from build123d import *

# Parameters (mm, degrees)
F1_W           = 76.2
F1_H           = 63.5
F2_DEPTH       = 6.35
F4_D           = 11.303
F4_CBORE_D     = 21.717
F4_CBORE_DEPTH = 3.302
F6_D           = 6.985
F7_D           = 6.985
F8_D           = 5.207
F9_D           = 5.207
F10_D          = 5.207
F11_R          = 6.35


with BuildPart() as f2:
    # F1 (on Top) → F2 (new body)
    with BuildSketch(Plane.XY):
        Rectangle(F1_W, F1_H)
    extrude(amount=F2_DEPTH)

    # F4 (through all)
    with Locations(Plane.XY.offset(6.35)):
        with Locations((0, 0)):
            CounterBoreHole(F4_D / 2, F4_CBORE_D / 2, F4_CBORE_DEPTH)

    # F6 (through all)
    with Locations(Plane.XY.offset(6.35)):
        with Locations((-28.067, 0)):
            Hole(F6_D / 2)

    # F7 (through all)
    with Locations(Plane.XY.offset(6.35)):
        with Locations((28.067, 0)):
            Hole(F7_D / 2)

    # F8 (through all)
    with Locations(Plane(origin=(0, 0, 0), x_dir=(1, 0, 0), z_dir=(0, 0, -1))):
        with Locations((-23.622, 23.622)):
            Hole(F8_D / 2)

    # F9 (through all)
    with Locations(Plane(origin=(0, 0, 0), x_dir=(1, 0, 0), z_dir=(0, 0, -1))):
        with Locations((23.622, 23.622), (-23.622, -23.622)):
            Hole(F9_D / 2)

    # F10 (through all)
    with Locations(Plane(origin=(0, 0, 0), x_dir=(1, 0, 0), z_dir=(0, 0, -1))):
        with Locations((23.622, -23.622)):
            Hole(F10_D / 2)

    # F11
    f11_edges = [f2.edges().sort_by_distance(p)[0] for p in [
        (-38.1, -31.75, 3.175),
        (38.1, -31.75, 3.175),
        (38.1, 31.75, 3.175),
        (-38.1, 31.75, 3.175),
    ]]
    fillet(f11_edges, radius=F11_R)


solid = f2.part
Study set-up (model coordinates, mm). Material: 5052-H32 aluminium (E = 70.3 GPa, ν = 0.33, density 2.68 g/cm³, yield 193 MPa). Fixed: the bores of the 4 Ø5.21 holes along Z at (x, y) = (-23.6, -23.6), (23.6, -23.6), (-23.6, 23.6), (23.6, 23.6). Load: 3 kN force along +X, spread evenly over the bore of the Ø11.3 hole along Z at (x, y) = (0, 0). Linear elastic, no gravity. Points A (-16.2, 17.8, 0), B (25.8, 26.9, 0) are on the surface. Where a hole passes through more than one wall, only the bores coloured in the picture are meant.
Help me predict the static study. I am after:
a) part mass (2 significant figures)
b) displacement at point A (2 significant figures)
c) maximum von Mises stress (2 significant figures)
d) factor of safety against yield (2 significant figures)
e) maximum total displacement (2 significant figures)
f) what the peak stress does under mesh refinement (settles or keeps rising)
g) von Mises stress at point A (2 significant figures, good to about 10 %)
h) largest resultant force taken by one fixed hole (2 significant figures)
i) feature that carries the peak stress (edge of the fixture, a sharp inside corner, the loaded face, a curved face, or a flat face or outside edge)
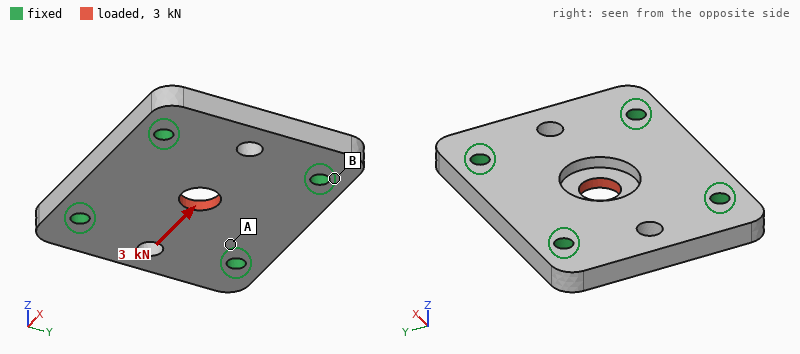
75 g
1.1 µm
50 MPa
3.9
6.9 µm
settles
9.7 MPa
800 N
the loaded face
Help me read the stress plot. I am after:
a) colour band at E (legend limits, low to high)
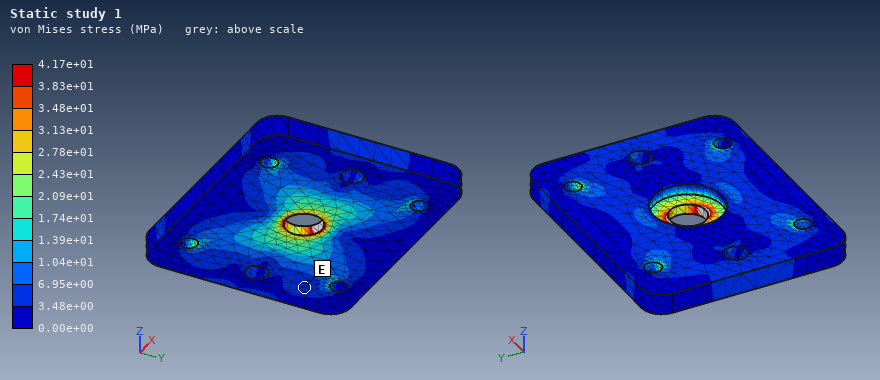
3.48e+00 to 6.95e+00 MPa
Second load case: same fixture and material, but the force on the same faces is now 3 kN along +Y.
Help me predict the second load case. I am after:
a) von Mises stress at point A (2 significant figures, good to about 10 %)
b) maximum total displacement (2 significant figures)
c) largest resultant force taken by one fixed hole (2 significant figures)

11 MPa
7.3 µm
840 N
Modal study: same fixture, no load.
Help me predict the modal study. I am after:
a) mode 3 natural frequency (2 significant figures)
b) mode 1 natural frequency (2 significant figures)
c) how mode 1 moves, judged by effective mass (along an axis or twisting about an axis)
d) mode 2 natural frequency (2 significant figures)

13 kHz
10 kHz
along Z
13 kHz
